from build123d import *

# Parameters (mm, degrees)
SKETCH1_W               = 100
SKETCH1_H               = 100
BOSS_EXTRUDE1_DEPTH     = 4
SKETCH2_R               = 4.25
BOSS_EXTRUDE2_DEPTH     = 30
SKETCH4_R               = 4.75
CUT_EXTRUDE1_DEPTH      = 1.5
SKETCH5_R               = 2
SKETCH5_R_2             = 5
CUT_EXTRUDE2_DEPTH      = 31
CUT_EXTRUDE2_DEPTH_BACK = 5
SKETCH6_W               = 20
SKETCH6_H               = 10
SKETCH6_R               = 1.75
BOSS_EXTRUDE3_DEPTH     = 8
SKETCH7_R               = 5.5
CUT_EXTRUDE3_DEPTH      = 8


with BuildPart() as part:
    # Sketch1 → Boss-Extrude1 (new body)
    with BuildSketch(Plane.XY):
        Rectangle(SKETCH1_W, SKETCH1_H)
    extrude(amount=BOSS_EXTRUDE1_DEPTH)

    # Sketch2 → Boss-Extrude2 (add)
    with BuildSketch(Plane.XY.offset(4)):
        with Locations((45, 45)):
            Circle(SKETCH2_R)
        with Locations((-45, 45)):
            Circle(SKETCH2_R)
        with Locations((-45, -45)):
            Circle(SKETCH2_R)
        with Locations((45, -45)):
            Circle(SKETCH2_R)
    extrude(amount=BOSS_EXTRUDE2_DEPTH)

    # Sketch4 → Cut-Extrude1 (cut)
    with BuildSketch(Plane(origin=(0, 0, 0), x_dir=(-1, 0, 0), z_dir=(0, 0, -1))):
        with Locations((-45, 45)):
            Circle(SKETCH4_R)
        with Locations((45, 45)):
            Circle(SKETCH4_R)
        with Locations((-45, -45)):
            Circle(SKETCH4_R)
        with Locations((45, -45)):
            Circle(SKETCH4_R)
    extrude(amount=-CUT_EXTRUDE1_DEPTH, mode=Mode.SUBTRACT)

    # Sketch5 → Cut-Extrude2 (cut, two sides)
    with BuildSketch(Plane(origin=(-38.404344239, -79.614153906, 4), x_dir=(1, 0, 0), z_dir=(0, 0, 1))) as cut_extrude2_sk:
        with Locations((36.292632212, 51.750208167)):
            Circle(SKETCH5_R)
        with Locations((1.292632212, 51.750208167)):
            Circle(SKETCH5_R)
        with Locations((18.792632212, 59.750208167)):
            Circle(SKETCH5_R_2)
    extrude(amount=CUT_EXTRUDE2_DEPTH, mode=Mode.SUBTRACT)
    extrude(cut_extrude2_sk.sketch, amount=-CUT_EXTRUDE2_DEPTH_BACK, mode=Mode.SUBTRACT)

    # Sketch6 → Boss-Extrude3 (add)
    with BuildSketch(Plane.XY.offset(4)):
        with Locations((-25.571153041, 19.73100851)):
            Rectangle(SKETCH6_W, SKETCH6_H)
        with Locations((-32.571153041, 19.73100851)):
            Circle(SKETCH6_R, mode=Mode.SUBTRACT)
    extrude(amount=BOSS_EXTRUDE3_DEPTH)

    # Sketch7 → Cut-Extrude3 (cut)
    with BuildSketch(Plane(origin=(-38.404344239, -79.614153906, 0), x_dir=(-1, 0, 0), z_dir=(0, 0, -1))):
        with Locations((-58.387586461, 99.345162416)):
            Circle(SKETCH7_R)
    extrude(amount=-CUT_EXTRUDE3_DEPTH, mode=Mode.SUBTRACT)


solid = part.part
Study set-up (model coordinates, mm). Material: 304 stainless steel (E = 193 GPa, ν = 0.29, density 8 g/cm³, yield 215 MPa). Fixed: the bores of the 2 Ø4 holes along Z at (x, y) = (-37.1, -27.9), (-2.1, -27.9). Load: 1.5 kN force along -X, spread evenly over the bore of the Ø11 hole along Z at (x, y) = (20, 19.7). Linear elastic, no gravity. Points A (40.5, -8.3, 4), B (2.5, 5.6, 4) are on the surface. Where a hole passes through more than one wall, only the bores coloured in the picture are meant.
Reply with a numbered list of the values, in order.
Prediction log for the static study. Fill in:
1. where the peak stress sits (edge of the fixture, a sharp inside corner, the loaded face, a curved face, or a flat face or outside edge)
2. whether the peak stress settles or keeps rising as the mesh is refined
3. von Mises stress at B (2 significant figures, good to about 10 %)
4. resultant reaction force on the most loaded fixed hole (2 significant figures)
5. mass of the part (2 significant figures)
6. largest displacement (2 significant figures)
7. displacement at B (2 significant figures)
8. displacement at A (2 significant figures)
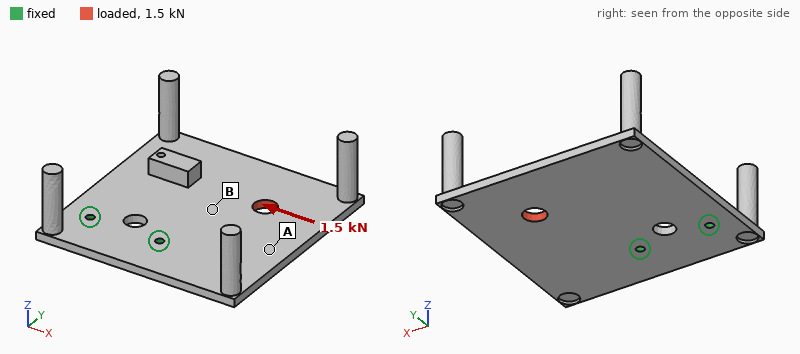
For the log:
1. edge of the fixture
2. keeps rising
3. 11 MPa
4. 2.1 kN
5. 380 g
6. 21 µm
7. 8.5 µm
8. 12 µm
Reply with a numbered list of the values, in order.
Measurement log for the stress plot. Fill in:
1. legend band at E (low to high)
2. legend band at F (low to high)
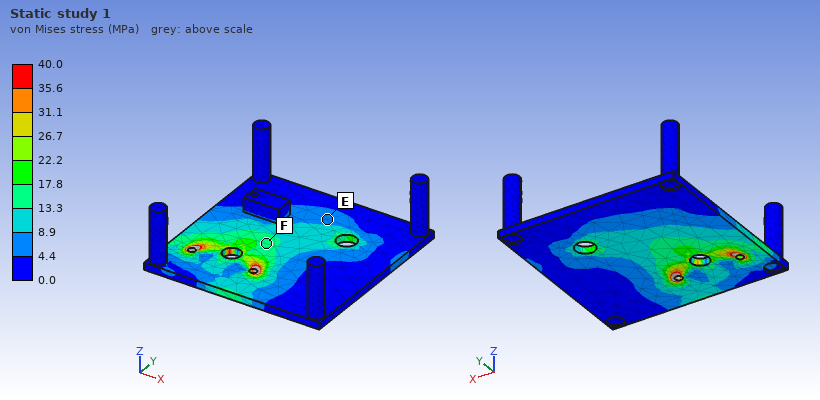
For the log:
1. 4.4 to 8.9 MPa
2. 13.3 to 17.8 MPa
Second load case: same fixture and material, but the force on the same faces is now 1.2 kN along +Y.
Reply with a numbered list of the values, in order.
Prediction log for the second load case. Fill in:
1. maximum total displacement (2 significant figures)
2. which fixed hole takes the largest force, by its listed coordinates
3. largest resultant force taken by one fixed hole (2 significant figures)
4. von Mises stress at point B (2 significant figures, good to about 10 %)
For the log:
1. 12 µm
2. (-2.1, -27.9)
3. 1.9 kN
4. 8.2 MPa
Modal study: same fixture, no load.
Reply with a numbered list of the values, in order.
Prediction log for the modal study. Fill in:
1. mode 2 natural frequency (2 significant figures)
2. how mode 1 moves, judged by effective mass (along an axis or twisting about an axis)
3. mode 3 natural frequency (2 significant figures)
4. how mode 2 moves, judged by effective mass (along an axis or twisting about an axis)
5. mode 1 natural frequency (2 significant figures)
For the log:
1. 620 Hz
2. along Z
3. 1000 Hz
4. twisting about Y
5. 360 Hz
